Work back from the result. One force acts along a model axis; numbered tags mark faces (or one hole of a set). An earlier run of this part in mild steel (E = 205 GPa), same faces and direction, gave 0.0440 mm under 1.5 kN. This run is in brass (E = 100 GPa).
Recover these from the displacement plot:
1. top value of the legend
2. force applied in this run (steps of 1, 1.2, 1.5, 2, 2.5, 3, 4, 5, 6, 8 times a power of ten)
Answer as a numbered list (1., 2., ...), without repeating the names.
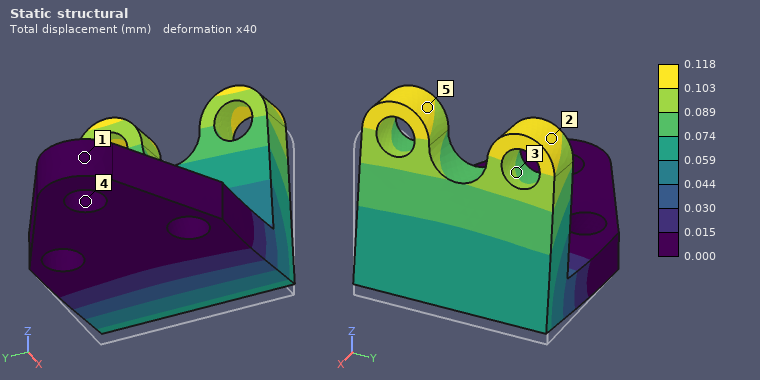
1. 0.118 mm
2. 2 kN
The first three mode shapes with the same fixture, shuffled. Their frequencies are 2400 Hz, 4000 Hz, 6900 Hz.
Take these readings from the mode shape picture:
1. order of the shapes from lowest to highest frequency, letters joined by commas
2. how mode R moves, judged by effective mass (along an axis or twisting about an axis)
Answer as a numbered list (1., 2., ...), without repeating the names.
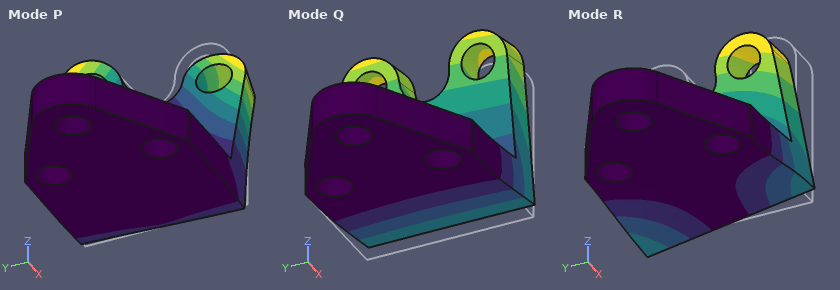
1. Q, R, P
2. along Y
